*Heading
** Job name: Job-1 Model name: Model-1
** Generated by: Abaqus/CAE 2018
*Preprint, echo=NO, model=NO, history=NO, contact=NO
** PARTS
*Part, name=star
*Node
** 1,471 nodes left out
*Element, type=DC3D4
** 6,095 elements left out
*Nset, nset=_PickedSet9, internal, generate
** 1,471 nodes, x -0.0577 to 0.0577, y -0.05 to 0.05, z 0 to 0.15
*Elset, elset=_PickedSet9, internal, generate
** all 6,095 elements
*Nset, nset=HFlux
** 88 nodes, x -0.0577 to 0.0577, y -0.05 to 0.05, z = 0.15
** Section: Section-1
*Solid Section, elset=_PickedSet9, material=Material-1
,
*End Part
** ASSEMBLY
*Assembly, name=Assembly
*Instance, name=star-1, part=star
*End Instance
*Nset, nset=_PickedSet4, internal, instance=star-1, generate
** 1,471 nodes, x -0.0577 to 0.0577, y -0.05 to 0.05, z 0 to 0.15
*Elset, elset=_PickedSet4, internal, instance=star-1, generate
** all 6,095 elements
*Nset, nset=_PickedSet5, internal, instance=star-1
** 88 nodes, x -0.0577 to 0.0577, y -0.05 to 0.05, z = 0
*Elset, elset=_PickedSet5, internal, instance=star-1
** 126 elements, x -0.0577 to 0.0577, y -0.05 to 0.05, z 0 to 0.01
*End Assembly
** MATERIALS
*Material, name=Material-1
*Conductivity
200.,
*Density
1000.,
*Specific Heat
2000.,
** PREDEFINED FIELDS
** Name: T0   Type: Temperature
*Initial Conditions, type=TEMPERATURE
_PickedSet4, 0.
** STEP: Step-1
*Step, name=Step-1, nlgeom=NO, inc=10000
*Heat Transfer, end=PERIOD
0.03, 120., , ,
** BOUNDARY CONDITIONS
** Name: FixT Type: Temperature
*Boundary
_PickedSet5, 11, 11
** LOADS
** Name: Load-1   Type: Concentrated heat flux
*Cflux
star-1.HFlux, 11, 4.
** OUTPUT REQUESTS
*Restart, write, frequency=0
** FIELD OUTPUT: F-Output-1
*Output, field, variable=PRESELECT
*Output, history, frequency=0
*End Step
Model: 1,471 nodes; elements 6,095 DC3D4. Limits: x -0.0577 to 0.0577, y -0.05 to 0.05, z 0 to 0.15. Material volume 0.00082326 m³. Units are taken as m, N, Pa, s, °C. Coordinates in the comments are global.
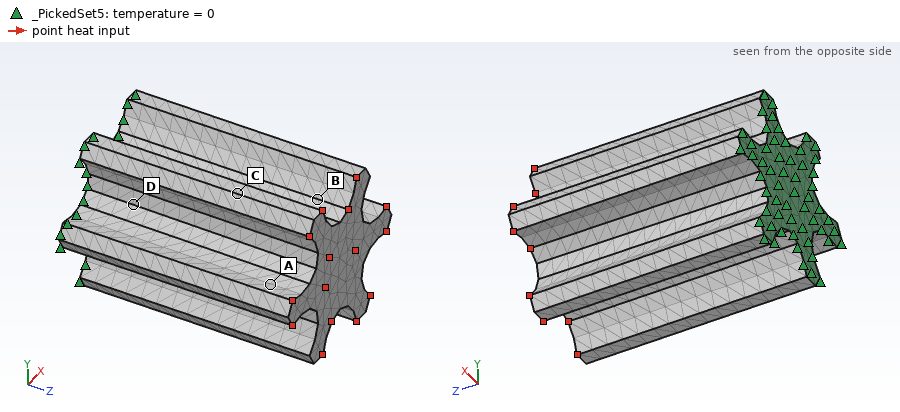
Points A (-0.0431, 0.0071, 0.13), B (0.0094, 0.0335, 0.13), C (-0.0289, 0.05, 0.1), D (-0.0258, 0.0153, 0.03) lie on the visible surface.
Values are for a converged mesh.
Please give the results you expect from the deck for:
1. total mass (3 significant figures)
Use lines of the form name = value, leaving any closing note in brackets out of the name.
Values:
total mass = 0.823 kg
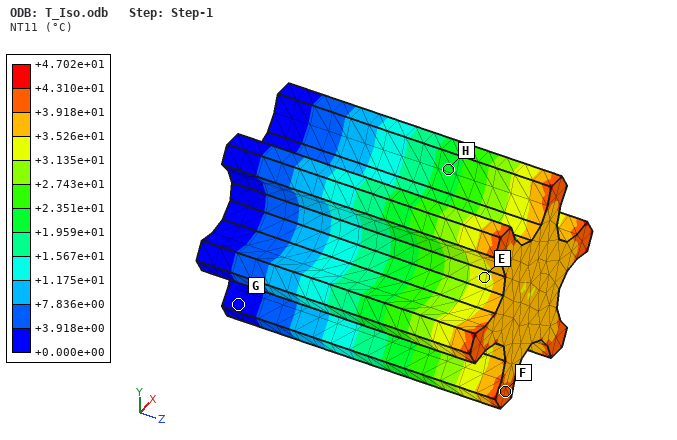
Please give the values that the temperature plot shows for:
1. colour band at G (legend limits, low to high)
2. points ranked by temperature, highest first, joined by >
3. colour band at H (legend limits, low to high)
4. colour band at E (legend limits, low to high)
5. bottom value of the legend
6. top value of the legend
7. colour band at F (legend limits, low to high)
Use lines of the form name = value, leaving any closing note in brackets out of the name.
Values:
colour band at G = +0.000e+00 to +3.918e+00 °C
points ranked by temperature, highest first, joined by > = F > E > H > G
colour band at H = +1.959e+01 to +2.351e+01 °C
colour band at E = +3.135e+01 to +3.526e+01 °C
bottom value of the legend = +0.000e+00 °C
top value of the legend = +4.702e+01 °C
colour band at F = +3.918e+01 to +4.310e+01 °C
